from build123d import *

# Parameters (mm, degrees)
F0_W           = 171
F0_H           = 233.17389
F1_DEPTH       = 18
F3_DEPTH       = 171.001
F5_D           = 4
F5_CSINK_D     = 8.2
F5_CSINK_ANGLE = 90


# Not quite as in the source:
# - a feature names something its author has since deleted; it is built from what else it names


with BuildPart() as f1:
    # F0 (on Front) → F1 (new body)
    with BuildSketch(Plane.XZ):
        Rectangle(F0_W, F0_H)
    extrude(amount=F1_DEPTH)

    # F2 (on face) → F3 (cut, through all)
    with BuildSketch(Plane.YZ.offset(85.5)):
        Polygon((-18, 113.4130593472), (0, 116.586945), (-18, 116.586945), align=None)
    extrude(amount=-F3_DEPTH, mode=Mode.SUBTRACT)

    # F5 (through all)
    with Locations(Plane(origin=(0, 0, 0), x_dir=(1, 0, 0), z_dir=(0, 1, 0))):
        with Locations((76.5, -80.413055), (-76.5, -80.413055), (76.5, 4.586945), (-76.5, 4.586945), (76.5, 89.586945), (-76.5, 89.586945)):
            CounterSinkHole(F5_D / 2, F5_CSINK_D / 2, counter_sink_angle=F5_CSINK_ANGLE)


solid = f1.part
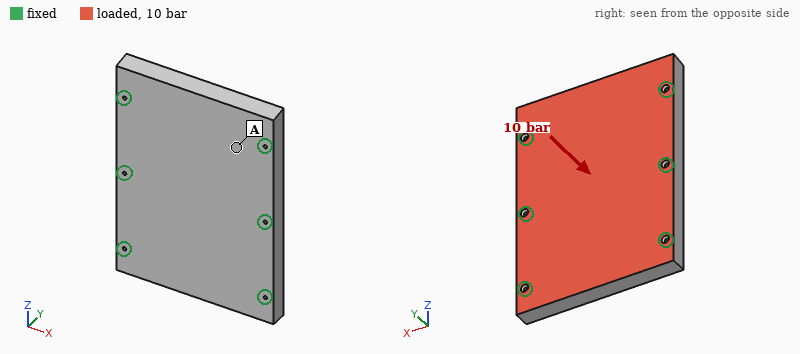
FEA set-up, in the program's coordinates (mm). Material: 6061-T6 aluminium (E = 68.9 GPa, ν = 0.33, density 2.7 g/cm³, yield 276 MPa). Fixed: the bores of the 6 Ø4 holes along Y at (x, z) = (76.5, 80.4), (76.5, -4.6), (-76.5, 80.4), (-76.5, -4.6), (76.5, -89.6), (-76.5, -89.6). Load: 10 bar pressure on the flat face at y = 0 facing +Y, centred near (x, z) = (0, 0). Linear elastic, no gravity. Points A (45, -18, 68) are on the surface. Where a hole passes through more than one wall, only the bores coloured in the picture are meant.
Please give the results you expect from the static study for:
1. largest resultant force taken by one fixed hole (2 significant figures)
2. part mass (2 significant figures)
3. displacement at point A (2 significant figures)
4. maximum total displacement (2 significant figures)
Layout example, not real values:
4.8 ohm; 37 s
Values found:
7.0 kN; 1.9 kg; 0.063 mm; 0.13 mm
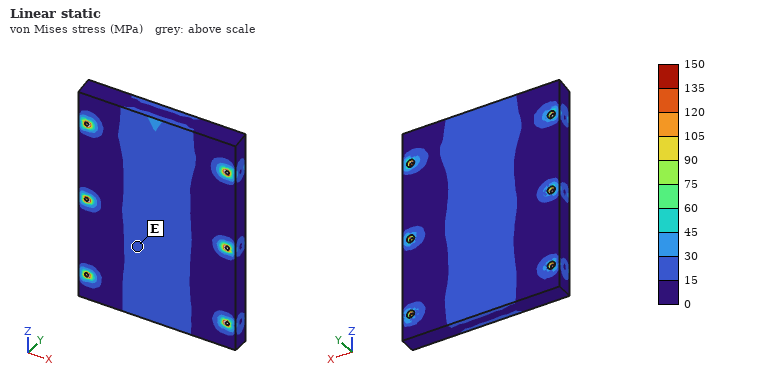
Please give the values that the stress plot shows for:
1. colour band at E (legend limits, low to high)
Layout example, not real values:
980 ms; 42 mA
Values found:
15 to 30 MPa
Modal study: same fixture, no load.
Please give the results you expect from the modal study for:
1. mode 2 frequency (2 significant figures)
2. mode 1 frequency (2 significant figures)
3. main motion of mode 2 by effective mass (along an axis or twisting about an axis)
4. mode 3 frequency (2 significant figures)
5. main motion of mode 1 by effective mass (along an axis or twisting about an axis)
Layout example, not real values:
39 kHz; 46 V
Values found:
2900 Hz; 2500 Hz; twisting about X; 4000 Hz; along Y
